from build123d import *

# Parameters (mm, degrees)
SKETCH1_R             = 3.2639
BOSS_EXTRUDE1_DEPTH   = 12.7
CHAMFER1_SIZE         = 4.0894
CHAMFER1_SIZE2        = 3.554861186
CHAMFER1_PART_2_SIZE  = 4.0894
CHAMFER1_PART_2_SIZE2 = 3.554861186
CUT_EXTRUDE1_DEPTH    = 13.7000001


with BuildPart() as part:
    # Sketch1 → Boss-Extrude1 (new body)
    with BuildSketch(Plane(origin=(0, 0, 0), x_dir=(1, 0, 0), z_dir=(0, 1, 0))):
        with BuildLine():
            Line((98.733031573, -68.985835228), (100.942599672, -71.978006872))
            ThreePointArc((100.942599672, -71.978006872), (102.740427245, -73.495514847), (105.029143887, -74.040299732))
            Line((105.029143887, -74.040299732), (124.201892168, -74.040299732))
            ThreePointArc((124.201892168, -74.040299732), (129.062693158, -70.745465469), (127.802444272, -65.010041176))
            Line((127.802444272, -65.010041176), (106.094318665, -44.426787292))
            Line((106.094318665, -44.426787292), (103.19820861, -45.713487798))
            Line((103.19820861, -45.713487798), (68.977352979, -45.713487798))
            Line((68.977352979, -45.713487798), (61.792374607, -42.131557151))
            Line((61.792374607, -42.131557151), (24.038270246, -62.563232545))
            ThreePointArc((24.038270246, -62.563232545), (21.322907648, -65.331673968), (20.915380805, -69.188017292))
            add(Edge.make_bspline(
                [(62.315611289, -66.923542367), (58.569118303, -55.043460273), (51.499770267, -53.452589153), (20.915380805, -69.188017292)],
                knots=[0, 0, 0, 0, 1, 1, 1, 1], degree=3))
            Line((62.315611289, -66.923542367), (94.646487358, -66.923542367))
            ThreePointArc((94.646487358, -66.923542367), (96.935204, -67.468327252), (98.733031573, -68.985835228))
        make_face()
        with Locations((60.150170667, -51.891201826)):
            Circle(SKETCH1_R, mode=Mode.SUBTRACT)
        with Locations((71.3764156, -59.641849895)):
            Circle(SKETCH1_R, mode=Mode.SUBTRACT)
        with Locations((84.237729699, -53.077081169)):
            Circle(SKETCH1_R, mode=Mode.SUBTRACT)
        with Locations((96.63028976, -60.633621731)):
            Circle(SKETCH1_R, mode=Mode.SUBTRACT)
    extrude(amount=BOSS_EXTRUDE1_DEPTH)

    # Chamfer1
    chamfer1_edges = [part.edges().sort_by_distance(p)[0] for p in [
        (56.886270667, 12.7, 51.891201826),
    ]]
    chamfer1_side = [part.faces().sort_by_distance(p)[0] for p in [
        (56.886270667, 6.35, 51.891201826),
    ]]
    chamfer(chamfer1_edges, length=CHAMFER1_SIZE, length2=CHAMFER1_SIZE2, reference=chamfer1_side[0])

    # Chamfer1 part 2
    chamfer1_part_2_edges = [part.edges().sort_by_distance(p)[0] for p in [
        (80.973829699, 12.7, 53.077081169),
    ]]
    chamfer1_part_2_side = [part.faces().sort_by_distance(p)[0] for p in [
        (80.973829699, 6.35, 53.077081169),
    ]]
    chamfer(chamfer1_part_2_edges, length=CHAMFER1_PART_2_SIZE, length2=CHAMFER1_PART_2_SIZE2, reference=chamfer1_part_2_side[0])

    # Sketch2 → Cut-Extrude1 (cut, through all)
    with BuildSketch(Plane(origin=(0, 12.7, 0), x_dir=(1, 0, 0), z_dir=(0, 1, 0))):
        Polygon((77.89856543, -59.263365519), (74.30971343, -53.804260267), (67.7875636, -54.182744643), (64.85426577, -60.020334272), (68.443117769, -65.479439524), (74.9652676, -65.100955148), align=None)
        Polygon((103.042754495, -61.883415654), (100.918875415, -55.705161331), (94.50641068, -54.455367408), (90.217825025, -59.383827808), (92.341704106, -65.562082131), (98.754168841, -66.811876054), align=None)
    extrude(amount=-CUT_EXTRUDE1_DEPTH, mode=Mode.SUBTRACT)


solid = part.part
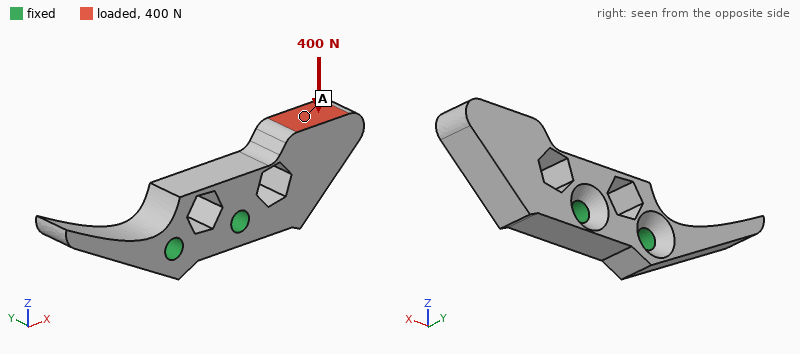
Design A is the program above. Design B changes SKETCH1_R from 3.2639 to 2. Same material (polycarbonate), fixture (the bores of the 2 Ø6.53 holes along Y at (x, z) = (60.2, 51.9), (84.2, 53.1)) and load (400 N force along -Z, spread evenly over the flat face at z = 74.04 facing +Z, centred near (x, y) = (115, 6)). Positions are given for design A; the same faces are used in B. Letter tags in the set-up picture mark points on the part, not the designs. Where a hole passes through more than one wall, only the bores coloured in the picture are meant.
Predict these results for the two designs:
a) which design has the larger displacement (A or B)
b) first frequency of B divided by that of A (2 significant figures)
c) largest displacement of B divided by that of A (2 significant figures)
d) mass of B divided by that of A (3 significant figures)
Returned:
B
0.95
1.2
1.04
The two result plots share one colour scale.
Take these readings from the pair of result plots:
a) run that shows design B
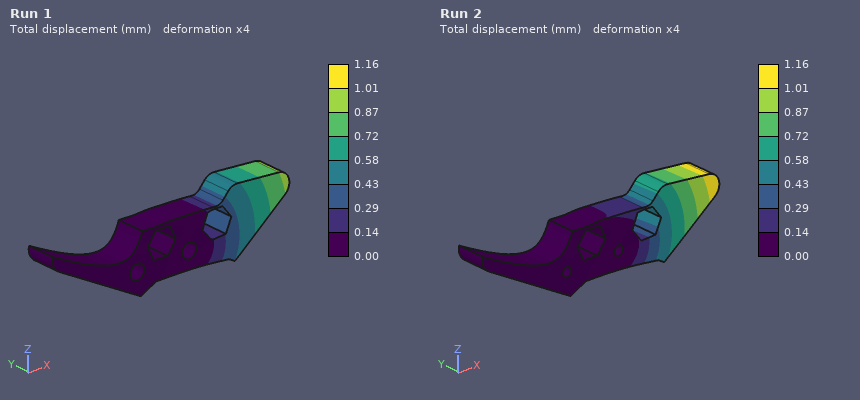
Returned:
Run 2
